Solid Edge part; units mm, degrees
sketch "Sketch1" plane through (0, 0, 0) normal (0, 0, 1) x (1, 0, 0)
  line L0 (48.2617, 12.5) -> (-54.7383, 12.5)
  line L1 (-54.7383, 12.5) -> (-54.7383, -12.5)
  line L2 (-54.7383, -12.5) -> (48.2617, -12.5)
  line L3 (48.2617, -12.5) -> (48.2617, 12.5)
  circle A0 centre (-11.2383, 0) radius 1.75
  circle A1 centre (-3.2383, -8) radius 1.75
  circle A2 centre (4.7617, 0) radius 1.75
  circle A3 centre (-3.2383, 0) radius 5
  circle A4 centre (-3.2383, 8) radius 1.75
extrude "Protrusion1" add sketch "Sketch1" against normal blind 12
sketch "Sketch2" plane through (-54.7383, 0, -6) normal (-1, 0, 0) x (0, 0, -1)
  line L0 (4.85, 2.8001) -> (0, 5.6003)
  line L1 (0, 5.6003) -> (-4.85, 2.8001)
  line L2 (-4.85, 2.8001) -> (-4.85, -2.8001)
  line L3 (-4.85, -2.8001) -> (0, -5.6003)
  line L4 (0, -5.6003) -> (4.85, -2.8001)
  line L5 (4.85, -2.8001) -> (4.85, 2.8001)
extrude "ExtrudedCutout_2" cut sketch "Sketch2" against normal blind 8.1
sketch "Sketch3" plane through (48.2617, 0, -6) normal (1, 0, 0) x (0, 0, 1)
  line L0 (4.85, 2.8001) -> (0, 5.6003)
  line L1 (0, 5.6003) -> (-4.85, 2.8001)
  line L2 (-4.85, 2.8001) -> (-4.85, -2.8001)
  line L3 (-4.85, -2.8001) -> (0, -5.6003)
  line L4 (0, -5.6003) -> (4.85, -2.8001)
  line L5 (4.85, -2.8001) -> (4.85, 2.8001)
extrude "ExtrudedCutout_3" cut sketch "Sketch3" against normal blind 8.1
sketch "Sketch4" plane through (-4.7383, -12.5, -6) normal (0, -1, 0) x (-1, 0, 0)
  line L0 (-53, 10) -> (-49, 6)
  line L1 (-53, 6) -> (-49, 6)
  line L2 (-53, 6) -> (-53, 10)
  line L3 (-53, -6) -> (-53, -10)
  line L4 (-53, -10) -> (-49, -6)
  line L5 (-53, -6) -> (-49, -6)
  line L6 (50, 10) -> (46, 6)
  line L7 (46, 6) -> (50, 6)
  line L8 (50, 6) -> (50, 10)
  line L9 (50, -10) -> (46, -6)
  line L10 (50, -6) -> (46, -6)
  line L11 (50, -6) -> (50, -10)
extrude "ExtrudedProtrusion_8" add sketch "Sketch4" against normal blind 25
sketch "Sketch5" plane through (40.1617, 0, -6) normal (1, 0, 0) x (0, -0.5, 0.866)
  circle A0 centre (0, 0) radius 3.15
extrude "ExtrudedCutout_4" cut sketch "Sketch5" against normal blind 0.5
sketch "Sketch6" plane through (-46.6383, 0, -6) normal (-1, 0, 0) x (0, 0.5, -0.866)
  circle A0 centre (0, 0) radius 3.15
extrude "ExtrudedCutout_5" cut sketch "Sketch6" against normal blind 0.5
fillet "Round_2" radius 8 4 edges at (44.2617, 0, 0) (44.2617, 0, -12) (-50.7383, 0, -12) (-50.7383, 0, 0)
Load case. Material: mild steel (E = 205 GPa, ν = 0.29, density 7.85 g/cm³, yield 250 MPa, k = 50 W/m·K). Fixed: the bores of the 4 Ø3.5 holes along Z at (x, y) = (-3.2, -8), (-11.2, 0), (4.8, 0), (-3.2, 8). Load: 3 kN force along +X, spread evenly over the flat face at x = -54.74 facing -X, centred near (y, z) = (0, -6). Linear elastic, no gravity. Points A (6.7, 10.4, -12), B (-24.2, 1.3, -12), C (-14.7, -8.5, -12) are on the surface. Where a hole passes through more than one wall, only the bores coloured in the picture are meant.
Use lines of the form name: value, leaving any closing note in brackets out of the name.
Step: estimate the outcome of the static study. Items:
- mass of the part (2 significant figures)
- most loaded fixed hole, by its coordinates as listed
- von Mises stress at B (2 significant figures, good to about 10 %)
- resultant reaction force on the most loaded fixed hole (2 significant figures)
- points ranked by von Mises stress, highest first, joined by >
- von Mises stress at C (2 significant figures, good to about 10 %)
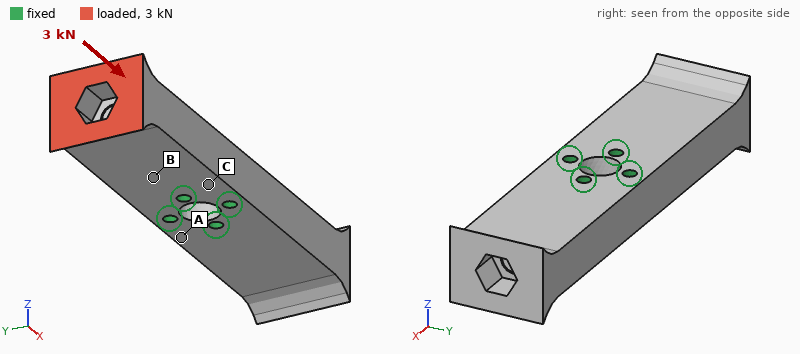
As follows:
mass of the part: 230 g
most loaded fixed hole, by its coordinates as listed: (-11.2, 0)
von Mises stress at B: 11 MPa
resultant reaction force on the most loaded fixed hole: 1.6 kN
points ranked by von Mises stress, highest first, joined by >: B > C > A
von Mises stress at C: 7.6 MPa
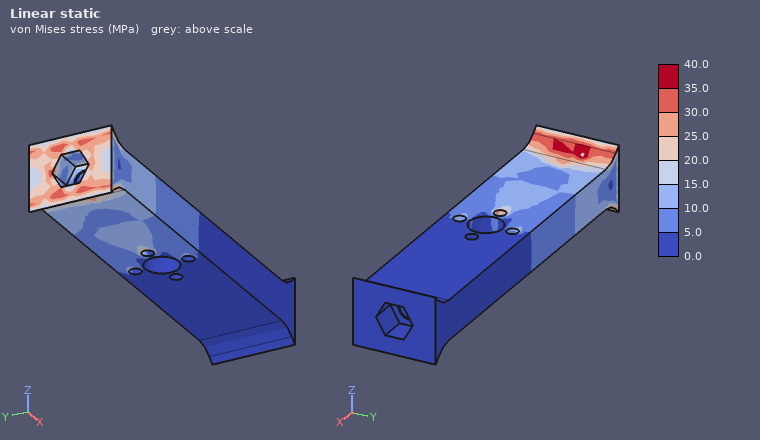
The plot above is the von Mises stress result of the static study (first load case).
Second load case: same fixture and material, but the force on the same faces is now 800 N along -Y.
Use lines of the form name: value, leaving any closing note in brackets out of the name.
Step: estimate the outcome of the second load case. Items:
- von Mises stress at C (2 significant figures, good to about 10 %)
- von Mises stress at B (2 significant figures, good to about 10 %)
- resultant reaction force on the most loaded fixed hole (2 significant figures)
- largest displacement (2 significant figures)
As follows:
von Mises stress at C: 17 MPa
von Mises stress at B: 7.0 MPa
resultant reaction force on the most loaded fixed hole: 1.7 kN
largest displacement: 13 µm
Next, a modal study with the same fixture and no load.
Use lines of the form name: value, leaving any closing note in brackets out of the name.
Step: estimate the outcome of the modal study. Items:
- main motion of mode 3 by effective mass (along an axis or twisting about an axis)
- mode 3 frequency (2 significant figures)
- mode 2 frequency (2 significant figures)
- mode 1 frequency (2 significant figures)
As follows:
main motion of mode 3 by effective mass: twisting about Z
mode 3 frequency: 7300 Hz
mode 2 frequency: 4600 Hz
mode 1 frequency: 4600 Hz
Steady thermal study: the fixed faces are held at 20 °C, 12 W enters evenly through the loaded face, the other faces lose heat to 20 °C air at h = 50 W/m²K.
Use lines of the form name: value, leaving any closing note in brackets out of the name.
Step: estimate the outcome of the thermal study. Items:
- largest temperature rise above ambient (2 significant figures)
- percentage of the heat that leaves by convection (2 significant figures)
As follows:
largest temperature rise above ambient: 34 K
percentage of the heat that leaves by convection: 26 %
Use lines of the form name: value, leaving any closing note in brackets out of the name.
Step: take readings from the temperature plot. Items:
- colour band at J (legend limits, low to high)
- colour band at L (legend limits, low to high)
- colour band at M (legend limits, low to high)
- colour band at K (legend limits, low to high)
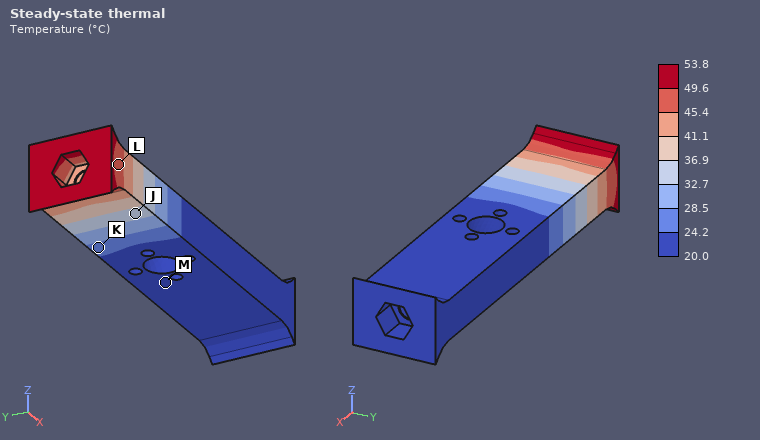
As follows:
colour band at J: 32.7 to 36.9 °C
colour band at L: 45.4 to 49.6 °C
colour band at M: 20.0 to 24.2 °C
colour band at K: 24.2 to 28.5 °C
